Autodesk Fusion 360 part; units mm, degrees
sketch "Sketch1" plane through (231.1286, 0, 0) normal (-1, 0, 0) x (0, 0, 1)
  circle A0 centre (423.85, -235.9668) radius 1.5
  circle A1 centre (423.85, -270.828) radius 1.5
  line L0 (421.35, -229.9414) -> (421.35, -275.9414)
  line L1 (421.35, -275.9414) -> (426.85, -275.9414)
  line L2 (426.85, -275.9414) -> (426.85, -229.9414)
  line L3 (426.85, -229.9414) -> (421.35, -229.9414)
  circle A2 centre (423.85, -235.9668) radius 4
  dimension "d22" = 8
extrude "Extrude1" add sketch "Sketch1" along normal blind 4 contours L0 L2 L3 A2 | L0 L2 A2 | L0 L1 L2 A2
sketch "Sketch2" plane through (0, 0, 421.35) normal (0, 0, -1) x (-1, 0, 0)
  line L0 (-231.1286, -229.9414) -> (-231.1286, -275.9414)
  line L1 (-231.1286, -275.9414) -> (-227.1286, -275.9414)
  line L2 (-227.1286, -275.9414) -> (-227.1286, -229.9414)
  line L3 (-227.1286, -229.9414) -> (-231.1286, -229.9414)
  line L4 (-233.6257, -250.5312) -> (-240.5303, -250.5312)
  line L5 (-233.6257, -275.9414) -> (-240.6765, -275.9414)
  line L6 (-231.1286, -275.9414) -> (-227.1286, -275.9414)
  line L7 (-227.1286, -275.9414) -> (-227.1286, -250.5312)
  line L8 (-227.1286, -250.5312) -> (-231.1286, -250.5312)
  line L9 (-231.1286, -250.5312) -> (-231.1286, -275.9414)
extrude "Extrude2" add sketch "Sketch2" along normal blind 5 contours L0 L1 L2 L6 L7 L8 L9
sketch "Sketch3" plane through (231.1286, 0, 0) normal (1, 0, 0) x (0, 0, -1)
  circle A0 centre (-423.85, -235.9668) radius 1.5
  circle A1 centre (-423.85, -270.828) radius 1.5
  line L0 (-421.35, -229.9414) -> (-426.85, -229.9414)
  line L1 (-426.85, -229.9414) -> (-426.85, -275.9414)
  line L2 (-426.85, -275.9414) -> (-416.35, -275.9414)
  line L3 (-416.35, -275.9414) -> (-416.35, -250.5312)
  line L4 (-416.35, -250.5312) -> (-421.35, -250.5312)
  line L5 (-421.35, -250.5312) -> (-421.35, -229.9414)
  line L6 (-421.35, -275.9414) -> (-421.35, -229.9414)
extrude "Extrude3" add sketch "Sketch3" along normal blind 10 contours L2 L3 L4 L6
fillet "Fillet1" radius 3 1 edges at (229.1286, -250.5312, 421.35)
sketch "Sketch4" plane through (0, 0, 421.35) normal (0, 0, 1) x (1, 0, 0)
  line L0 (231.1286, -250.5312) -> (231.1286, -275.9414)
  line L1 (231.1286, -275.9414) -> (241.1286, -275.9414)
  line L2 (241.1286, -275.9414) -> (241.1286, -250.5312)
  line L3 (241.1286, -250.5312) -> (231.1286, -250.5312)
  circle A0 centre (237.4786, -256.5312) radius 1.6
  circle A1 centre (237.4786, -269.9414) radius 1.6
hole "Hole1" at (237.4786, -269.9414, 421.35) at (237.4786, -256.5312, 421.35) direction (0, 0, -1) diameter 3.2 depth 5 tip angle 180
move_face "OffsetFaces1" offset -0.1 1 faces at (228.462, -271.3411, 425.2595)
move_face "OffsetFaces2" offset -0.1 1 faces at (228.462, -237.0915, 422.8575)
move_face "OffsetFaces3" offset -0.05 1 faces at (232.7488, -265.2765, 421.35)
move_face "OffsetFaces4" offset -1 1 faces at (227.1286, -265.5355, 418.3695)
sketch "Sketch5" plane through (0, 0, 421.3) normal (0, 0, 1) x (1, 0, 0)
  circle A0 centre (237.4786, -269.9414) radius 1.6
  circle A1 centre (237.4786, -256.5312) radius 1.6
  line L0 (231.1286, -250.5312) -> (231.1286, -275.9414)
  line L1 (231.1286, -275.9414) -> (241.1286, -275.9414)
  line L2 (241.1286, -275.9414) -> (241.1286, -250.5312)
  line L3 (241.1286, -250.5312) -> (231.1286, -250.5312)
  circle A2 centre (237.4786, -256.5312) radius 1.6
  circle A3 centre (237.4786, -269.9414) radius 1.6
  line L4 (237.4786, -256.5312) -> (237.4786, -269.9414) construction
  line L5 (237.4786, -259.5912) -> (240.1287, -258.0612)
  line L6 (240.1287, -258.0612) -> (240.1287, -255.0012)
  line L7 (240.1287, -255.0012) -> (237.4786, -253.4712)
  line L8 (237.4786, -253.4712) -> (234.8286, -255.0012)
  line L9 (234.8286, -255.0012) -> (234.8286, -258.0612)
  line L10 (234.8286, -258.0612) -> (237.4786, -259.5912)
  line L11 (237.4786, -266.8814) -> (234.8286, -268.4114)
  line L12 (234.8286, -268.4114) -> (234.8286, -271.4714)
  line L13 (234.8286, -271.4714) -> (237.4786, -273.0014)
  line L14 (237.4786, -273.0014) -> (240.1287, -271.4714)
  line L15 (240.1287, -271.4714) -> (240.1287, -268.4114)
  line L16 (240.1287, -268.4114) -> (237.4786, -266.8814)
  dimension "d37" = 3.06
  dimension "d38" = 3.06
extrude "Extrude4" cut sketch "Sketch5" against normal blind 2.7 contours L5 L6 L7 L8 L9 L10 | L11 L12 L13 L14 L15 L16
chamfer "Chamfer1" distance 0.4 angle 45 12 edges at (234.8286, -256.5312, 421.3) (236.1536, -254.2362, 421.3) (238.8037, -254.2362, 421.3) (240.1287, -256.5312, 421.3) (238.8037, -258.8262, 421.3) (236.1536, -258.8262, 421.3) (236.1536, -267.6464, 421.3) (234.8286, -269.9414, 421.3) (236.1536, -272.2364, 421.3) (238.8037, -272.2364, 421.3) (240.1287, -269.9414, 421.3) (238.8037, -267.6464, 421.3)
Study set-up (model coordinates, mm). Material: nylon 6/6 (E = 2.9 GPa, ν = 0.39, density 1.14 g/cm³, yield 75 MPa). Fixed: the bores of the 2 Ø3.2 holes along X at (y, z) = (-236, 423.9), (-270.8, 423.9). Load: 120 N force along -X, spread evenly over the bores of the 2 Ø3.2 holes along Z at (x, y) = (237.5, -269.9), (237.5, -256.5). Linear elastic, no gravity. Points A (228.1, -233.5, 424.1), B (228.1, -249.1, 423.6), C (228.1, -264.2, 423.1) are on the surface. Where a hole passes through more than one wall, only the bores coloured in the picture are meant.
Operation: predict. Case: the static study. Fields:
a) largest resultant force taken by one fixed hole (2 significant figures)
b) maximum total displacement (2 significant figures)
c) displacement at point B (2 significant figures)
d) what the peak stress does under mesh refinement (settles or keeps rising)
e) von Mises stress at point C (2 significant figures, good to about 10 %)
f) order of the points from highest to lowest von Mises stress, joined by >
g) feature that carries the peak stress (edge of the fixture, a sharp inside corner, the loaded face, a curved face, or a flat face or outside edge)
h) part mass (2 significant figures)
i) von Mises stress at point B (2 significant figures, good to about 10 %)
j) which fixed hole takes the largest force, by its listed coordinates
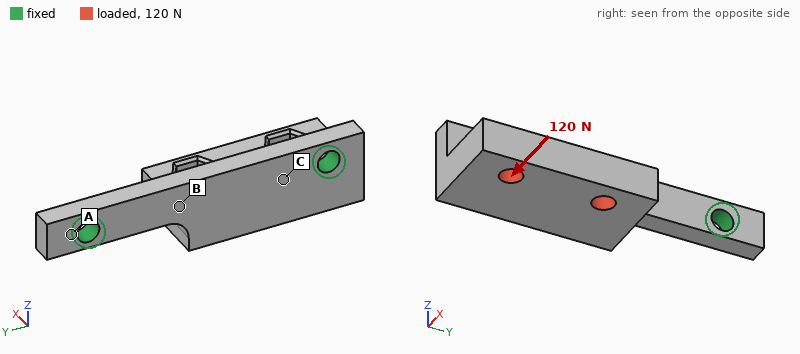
100 N
0.51 mm
0.14 mm
keeps rising
8.1 MPa
B > C > A
edge of the fixture
2.5 g
14 MPa
(-270.8, 423.9)
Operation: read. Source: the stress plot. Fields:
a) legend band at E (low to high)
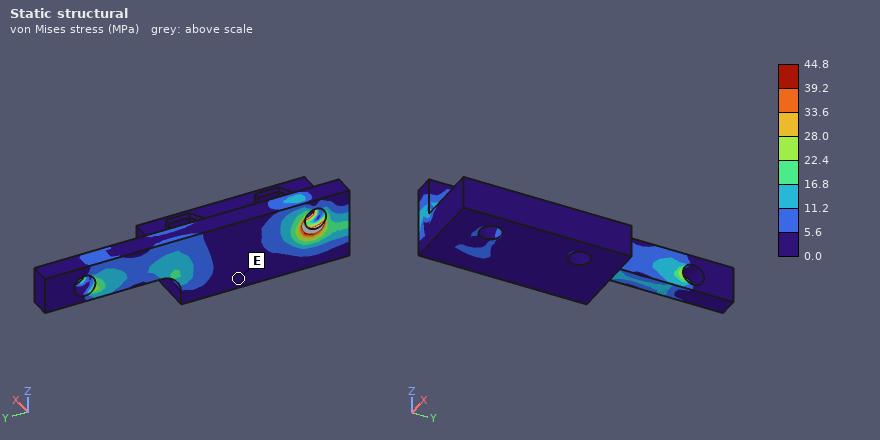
0.0 to 5.6 MPa
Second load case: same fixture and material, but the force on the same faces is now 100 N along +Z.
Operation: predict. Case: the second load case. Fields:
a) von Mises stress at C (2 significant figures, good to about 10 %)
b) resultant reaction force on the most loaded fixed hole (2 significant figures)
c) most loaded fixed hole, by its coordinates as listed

12 MPa
82 N
(-270.8, 423.9)
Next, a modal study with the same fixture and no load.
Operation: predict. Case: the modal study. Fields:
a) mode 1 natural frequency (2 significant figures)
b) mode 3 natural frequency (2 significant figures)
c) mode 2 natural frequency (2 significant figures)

2300 Hz
5100 Hz
3200 Hz
